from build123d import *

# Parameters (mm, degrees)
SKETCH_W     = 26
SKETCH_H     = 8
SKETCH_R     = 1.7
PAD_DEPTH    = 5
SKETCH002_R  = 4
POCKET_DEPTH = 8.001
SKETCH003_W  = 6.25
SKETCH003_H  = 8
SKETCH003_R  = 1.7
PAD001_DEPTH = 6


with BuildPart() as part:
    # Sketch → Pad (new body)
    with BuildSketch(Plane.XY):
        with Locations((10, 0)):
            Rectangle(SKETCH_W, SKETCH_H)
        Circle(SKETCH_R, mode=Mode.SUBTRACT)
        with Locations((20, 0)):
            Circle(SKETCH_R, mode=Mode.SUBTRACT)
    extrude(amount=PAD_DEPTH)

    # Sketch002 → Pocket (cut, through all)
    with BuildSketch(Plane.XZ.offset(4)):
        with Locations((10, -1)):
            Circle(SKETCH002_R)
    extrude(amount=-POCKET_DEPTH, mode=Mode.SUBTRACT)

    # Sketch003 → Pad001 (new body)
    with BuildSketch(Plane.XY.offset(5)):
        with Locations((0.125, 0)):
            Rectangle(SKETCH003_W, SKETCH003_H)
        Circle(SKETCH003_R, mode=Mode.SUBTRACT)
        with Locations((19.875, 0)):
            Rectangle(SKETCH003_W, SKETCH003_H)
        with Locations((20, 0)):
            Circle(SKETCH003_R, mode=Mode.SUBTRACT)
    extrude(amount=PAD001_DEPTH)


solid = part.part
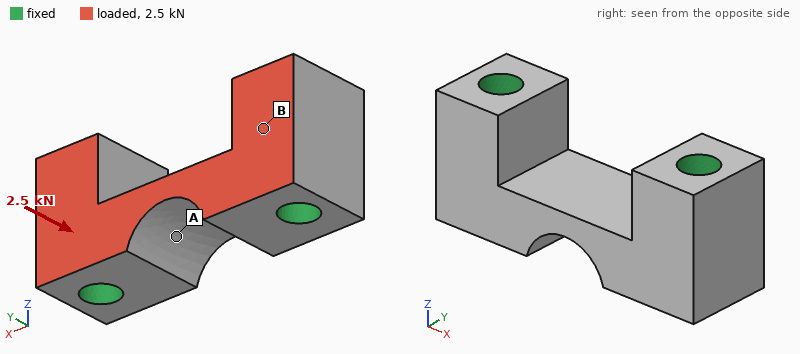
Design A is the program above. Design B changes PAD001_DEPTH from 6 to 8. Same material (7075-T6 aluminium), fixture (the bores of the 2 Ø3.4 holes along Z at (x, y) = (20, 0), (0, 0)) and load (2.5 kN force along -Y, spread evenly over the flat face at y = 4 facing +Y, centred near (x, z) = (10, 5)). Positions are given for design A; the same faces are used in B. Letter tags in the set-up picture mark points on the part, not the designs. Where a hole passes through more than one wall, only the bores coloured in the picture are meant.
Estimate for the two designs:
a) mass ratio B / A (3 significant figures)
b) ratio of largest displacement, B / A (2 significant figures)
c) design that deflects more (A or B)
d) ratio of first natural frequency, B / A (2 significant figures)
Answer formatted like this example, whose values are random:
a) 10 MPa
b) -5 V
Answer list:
a) 1.13
b) 0.88
c) A
d) 1.0
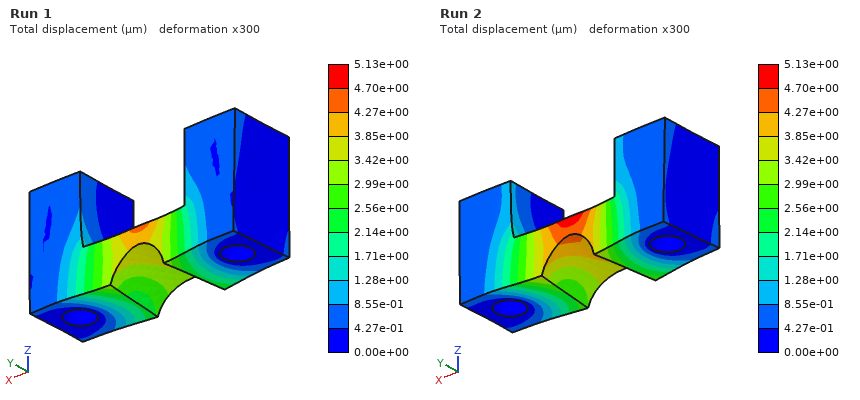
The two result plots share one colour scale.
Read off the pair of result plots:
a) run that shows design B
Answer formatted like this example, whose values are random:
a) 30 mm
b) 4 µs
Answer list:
a) Run 1
